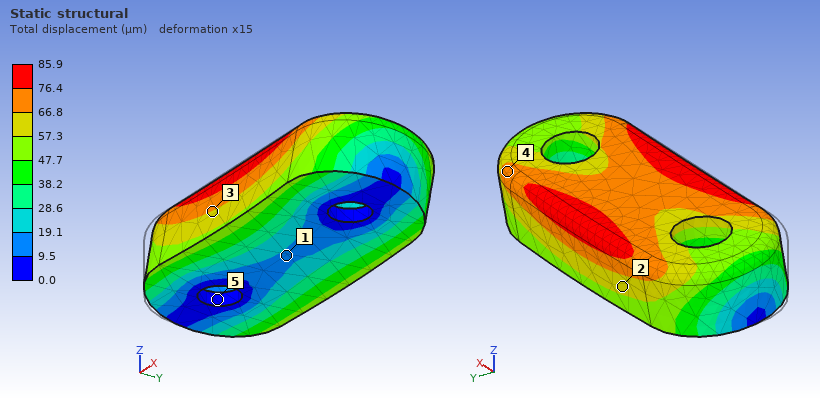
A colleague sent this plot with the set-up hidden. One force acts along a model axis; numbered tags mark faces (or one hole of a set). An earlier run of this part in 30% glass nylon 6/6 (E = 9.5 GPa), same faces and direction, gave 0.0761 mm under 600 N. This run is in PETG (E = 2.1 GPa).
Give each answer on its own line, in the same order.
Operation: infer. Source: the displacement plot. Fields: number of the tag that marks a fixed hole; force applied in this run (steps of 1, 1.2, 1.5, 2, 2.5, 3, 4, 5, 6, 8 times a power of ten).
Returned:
5
150 N
